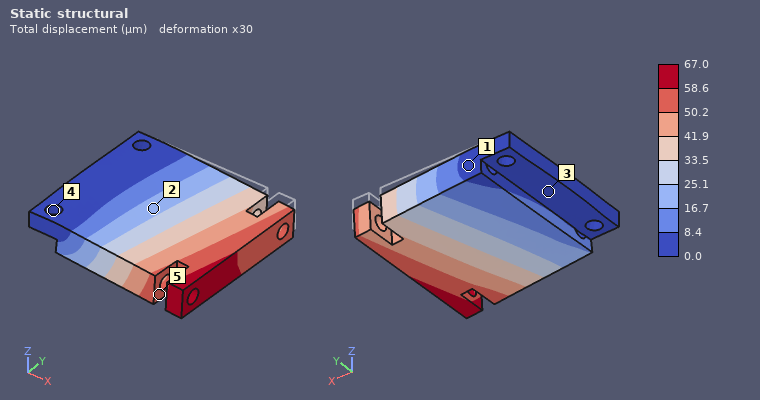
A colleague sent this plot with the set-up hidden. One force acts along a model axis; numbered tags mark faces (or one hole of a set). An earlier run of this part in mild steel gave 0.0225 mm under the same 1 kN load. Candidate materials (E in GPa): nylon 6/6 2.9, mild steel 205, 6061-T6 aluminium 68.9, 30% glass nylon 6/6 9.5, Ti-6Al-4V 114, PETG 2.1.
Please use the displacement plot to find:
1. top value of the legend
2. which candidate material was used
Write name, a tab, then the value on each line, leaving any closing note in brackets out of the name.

top value of the legend	67.0 µm
which candidate material was used	6061-T6 aluminium
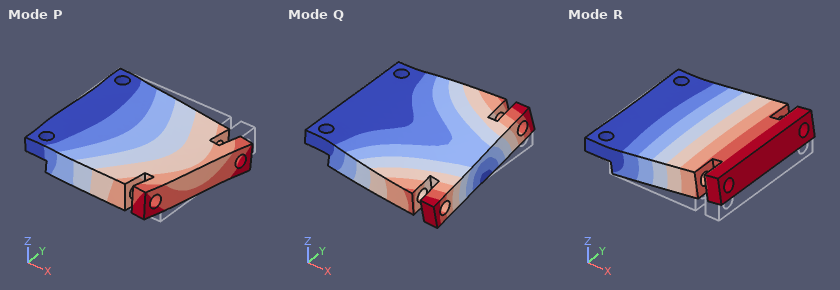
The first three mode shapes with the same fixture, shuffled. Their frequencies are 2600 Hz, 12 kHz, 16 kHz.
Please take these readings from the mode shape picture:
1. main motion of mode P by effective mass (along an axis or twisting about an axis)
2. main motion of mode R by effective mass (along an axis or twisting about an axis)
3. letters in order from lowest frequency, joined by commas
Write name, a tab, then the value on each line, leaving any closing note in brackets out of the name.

main motion of mode P by effective mass	along Y
main motion of mode R by effective mass	along Z
letters in order from lowest frequency, joined by commas	R, Q, P
